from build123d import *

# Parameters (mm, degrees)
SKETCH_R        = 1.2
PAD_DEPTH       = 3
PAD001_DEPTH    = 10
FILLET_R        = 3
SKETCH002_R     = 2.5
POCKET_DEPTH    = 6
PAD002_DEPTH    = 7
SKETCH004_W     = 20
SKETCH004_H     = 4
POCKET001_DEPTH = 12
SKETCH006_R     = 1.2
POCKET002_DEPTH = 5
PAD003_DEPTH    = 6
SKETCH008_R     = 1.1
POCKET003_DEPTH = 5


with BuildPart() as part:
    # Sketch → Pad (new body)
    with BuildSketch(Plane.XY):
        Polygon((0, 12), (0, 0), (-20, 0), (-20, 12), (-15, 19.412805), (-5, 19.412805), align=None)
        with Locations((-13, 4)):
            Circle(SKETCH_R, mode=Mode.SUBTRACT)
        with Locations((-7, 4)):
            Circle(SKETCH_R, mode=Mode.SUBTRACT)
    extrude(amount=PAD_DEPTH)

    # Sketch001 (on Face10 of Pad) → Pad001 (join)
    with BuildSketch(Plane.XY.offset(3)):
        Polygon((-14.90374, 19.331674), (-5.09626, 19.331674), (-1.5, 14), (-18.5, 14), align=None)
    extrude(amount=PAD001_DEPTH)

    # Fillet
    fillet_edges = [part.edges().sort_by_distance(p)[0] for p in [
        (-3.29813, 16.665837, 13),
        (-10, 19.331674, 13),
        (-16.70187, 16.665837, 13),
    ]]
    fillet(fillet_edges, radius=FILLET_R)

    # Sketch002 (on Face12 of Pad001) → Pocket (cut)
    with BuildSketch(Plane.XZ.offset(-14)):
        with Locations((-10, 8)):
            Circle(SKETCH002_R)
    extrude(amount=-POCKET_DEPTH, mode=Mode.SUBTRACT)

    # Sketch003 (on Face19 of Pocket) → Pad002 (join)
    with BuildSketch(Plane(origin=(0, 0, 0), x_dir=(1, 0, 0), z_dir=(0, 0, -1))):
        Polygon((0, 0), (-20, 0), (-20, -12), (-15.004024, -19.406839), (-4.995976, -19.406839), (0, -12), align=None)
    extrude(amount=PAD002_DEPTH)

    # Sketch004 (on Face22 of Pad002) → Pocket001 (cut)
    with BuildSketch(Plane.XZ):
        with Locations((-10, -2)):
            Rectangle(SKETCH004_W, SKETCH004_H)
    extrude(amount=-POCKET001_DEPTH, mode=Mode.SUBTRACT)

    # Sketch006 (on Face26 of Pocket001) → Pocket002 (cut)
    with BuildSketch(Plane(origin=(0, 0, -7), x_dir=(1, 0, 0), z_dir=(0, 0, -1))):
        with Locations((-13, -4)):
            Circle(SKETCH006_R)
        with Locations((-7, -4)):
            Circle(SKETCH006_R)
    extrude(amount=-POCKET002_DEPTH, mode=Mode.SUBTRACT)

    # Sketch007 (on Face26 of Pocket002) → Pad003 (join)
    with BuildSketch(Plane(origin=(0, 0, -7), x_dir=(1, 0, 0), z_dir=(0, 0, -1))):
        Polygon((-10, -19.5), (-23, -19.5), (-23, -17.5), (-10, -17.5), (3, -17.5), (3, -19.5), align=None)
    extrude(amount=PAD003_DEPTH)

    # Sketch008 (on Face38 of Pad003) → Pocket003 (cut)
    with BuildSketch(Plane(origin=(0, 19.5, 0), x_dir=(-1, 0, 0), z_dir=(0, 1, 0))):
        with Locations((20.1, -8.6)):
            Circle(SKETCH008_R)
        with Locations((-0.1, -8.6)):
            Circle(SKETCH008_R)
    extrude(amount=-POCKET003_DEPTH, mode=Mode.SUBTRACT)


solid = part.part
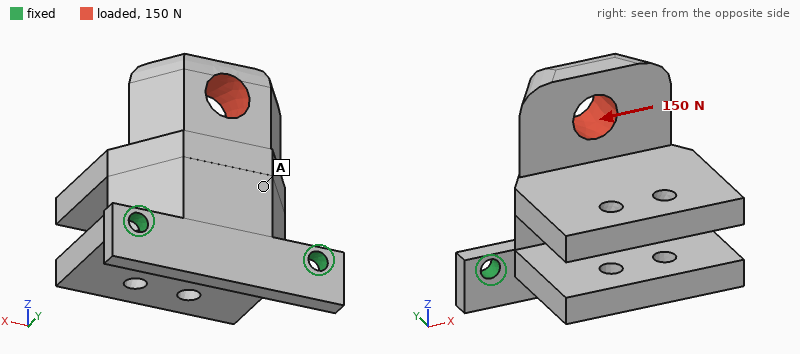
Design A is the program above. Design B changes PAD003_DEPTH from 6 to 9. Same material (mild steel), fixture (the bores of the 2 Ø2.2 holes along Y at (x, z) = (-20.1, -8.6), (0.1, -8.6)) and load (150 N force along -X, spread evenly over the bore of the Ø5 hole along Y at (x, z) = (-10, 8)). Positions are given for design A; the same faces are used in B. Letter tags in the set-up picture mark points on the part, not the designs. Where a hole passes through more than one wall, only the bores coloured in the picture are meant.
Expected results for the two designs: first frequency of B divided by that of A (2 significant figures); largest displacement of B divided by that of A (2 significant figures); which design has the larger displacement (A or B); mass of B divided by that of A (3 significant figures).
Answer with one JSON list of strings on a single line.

["1.0", "0.88", "A", "1.05"]
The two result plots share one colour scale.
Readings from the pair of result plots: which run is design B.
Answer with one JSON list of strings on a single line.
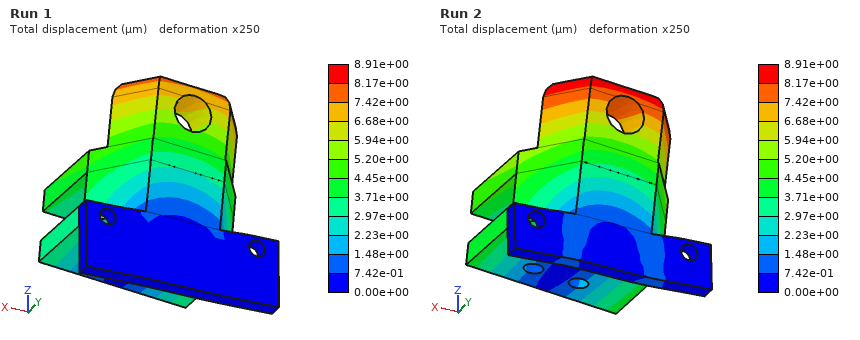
["Run 1"]
